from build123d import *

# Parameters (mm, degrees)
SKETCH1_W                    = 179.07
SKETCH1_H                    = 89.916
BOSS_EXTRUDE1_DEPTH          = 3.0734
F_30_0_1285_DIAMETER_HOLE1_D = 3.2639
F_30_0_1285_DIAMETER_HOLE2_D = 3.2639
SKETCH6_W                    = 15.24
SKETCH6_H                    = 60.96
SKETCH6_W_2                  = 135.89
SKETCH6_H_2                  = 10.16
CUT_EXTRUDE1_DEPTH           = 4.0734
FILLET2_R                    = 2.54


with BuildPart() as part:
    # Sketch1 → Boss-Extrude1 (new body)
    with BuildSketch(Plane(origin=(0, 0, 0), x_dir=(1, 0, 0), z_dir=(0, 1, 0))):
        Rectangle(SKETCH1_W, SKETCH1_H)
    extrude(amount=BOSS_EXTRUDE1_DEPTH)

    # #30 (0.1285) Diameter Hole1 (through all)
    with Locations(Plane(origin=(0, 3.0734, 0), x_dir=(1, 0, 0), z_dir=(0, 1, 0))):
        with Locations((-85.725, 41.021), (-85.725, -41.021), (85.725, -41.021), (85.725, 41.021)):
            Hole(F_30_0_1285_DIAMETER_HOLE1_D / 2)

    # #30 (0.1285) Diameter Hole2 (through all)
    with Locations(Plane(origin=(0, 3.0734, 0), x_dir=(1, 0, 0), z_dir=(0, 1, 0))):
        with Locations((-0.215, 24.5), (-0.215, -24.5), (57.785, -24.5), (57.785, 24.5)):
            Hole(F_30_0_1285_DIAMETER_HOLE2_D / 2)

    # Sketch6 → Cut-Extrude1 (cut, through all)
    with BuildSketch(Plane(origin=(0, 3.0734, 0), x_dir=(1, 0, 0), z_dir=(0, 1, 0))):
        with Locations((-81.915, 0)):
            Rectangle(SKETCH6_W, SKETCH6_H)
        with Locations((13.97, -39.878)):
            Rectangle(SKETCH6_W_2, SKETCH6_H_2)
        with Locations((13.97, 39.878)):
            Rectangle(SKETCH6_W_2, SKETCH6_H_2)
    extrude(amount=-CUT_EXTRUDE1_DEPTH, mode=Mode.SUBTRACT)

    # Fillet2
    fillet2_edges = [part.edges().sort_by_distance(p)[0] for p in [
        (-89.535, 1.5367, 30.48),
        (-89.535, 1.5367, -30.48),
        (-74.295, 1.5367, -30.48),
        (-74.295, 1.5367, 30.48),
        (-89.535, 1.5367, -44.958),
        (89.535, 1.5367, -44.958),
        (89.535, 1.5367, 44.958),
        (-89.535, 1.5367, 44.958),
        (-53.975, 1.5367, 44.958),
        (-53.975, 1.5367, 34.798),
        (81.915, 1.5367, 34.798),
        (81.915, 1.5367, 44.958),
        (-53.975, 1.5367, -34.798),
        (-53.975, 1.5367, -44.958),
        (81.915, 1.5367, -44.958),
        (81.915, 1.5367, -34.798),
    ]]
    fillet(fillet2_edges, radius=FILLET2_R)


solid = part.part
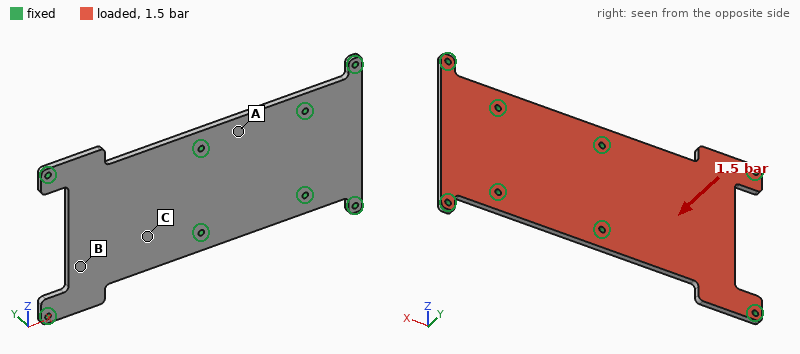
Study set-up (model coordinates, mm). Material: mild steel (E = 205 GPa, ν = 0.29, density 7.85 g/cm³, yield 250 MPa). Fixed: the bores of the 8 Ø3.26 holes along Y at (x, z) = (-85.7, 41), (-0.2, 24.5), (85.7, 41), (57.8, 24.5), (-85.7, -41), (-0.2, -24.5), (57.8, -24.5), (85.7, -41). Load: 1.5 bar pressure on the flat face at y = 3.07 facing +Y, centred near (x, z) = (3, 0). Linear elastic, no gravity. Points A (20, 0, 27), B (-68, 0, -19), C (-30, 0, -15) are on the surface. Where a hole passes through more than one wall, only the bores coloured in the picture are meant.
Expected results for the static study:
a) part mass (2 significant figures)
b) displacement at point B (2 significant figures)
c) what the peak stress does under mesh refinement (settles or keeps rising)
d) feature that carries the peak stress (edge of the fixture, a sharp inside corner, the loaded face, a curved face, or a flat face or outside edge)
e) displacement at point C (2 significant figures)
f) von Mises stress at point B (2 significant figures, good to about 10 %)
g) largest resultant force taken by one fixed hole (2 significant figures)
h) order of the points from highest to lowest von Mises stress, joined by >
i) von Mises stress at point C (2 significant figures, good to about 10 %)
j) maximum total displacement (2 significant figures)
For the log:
300 g
68 µm
keeps rising
edge of the fixture
61 µm
34 MPa
410 N
B > C > A
20 MPa
89 µm
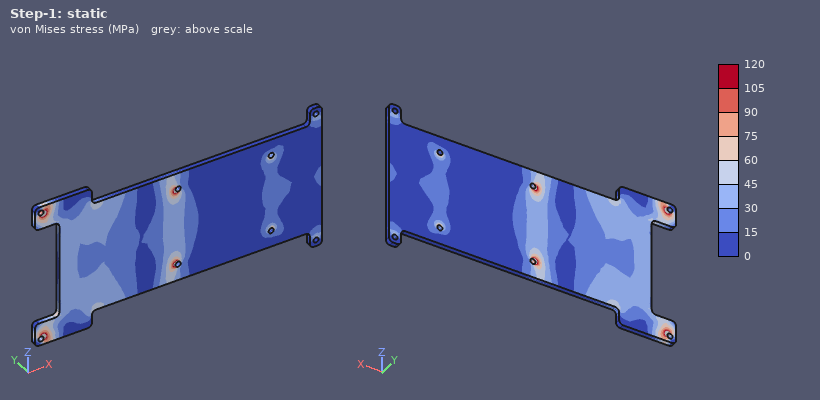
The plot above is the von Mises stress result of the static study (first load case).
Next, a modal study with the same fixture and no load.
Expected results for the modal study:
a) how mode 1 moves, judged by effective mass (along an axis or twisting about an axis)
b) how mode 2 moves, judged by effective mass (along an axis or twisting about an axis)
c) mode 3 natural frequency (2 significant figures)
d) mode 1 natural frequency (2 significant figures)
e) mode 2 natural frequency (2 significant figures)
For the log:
along Y
twisting about X
3300 Hz
1500 Hz
2600 Hz
